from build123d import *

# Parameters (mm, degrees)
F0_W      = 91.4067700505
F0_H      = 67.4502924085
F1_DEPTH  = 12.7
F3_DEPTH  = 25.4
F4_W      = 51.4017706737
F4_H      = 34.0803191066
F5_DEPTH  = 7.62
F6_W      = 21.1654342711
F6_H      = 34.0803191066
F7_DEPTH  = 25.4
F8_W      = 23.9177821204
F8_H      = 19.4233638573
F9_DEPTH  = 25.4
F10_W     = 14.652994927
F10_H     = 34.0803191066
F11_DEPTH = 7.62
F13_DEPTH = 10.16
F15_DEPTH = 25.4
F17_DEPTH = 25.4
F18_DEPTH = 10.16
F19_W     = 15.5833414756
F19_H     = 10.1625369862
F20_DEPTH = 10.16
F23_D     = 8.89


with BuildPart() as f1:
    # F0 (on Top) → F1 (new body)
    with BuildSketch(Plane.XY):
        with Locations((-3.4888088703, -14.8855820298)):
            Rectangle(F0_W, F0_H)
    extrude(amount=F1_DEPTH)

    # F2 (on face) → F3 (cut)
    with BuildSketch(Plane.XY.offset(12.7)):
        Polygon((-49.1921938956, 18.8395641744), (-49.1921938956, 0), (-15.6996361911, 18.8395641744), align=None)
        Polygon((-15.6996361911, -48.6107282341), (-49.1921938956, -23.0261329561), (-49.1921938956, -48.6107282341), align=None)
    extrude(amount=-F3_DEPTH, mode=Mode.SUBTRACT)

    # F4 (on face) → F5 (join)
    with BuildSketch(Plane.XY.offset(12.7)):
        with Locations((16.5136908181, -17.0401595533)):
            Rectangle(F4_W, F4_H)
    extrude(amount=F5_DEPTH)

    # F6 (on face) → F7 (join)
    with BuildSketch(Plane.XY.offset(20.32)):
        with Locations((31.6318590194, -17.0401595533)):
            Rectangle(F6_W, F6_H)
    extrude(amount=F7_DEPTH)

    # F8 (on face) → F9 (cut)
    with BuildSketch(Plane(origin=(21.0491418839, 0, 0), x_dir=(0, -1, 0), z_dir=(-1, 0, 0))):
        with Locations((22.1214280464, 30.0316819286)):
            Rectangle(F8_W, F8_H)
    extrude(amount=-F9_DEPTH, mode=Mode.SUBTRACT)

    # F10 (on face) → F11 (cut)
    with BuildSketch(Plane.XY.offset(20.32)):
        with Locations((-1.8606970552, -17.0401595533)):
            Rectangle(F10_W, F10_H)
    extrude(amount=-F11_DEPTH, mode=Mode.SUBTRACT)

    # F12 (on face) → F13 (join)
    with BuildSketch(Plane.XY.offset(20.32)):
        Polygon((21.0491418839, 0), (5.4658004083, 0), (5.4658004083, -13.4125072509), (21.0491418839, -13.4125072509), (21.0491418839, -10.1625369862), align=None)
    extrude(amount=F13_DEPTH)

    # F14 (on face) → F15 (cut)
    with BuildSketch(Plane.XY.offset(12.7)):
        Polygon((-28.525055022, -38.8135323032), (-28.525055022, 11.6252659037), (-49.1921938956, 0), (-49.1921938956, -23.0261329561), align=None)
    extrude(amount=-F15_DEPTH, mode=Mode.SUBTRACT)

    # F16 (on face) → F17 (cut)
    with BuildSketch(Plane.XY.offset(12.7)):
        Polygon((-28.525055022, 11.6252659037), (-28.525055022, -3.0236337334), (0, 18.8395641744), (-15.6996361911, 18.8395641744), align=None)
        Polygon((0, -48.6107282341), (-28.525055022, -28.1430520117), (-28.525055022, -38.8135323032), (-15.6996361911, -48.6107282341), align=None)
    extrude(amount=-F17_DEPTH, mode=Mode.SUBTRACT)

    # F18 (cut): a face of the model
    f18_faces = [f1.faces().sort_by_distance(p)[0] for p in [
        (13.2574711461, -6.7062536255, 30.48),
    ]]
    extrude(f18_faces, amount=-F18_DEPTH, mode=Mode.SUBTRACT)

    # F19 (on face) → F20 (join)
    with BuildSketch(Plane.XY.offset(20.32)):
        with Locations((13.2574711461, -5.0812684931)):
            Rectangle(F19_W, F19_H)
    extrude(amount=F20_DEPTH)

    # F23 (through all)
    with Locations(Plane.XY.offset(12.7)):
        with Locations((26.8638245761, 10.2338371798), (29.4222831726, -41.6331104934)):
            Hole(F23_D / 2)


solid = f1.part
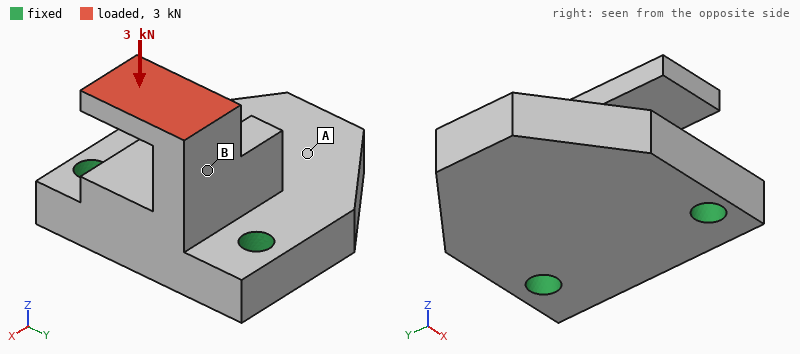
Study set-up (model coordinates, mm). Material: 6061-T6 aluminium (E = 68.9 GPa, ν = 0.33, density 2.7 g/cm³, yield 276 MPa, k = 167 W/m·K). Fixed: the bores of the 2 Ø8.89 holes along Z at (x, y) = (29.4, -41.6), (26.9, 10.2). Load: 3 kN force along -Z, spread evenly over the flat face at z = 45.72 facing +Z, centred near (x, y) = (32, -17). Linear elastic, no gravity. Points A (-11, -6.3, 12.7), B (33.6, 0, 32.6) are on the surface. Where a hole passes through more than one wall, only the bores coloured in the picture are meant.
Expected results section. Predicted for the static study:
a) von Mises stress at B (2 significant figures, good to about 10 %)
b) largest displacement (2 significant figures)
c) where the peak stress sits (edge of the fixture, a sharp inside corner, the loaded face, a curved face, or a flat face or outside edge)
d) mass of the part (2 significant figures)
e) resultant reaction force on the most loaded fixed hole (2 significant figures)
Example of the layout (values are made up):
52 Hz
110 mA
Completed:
73 MPa
0.43 mm
the loaded face
190 g
1.8 kN
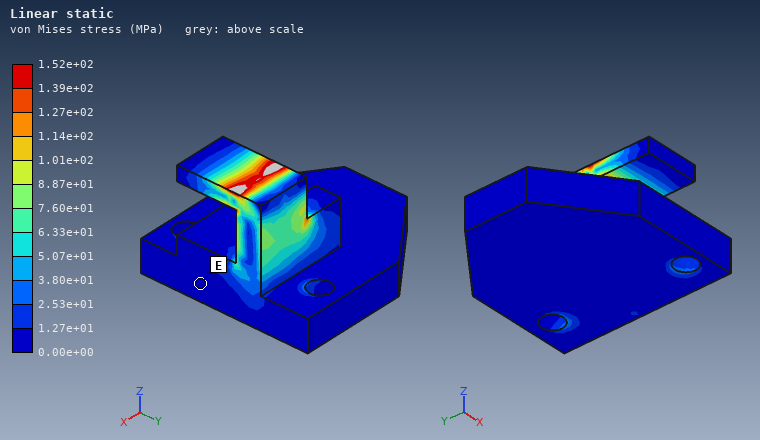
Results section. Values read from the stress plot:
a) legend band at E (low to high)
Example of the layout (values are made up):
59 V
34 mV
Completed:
0.00e+00 to 1.27e+01 MPa
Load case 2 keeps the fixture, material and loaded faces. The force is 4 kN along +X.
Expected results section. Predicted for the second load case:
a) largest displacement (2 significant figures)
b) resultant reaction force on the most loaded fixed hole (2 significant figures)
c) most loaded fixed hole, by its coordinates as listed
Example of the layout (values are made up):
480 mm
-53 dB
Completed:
0.38 mm
2.3 kN
(29.4, -41.6)
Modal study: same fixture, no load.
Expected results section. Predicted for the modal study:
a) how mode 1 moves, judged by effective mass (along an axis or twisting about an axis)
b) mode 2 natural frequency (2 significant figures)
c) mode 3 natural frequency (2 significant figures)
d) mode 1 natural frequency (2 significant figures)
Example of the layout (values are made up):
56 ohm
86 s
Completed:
along Z
4300 Hz
6300 Hz
3800 Hz
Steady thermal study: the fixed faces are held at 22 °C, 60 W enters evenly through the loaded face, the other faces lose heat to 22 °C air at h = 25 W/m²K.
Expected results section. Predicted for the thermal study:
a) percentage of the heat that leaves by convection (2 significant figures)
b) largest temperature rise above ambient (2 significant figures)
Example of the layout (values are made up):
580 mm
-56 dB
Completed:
6.6 %
74 K
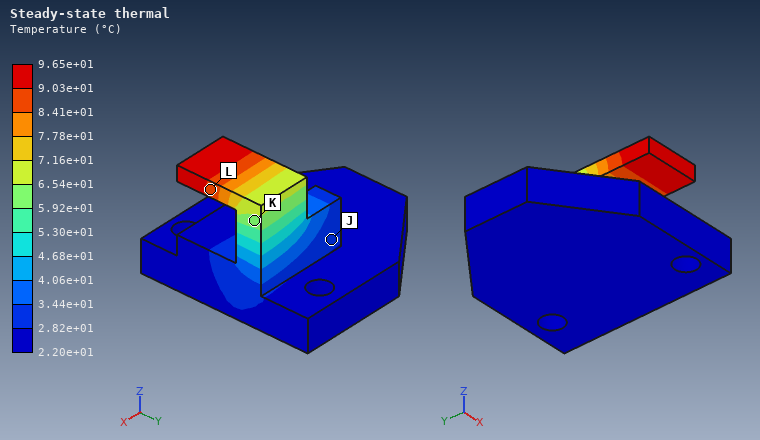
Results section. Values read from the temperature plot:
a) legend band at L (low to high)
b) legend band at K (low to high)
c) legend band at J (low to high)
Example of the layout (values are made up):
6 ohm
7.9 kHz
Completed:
8.41e+01 to 9.03e+01 °C
5.92e+01 to 6.54e+01 °C
2.82e+01 to 3.44e+01 °C
